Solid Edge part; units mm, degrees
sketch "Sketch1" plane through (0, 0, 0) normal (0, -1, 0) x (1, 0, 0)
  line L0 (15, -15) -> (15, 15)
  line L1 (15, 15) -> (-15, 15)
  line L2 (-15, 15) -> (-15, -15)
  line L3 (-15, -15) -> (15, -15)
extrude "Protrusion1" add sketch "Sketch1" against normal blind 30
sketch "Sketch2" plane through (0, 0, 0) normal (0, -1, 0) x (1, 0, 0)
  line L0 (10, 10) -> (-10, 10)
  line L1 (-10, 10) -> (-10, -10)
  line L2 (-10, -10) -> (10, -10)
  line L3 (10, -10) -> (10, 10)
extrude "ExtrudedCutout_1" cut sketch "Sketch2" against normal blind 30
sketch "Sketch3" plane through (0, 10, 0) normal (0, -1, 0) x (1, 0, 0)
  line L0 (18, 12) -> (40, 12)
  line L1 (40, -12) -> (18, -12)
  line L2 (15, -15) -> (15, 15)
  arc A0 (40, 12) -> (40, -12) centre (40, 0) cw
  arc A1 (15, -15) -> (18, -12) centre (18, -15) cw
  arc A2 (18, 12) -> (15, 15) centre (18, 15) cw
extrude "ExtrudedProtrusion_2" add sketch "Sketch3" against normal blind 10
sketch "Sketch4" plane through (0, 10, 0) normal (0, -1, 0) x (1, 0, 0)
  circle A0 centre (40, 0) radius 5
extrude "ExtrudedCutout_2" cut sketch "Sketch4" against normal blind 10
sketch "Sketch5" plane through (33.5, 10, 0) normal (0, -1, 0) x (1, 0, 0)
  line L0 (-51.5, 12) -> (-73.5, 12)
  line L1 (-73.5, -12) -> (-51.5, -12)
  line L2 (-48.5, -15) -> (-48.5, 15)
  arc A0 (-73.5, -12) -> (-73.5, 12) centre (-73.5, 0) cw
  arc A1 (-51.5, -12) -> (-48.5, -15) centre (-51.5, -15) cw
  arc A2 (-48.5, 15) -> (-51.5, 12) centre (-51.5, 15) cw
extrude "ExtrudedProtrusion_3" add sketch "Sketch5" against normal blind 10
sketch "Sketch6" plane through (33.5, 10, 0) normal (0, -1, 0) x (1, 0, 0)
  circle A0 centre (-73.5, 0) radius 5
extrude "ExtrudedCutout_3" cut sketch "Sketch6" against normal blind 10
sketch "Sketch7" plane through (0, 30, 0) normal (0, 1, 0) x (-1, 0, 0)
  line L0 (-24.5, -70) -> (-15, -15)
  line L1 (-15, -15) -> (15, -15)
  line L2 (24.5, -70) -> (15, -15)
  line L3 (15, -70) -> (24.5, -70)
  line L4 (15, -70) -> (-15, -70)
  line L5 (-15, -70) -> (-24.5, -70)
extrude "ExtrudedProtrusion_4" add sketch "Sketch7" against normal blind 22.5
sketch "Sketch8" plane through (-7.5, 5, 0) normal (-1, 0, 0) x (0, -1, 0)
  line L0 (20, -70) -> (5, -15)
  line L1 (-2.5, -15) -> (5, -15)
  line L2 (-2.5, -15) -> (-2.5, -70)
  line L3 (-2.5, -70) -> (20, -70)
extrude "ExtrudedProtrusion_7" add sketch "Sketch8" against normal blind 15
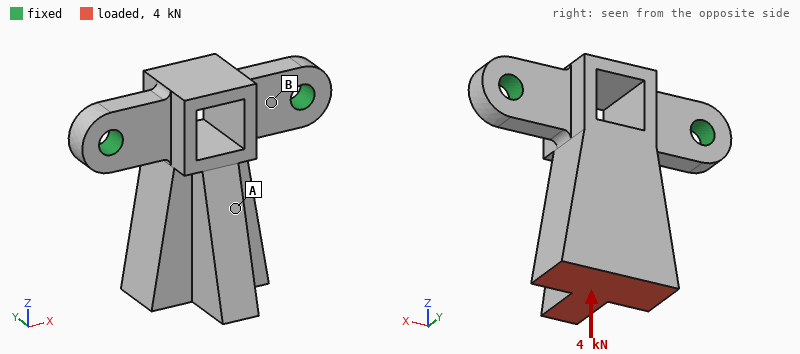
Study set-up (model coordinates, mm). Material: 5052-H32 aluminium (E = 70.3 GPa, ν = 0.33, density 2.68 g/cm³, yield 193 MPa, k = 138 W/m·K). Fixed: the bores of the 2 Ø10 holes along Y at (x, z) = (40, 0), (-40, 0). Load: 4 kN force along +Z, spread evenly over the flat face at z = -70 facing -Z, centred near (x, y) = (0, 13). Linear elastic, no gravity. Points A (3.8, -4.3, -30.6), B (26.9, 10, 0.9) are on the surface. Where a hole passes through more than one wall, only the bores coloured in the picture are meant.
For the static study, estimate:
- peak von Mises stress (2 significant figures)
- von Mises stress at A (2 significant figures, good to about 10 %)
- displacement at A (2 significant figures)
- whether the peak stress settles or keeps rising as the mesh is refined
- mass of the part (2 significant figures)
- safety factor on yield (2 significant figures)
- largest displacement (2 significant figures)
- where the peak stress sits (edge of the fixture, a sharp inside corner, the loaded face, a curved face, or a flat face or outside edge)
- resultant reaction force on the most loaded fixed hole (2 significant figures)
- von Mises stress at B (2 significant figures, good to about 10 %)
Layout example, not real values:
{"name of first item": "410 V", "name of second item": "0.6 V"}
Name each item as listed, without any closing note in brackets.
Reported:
{"peak von Mises stress": "72 MPa", "von Mises stress at A": "5.7 MPa", "displacement at A": "34 µm", "whether the peak stress settles or keeps rising as the mesh is refined": "settles", "mass of the part": "240 g", "safety factor on yield": "2.7", "largest displacement": "56 µm", "where the peak stress sits": "a curved face", "resultant reaction force on the most loaded fixed hole": "2.1 kN", "von Mises stress at B": "28 MPa"}
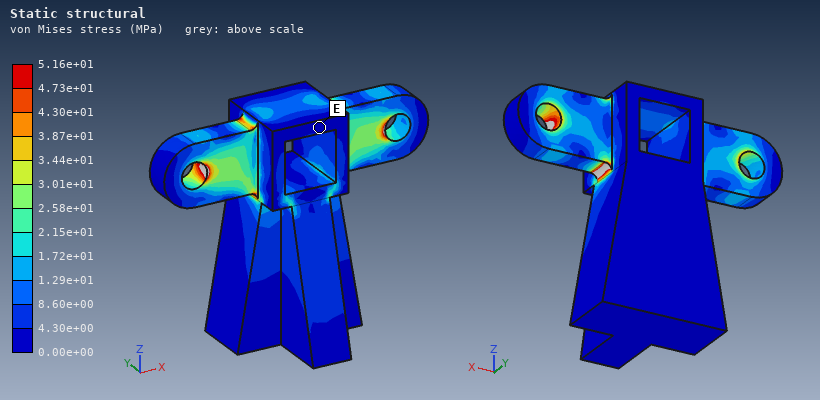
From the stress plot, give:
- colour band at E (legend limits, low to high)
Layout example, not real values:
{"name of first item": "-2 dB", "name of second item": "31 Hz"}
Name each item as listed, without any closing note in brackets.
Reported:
{"colour band at E": "0.00e+00 to 4.30e+00 MPa"}
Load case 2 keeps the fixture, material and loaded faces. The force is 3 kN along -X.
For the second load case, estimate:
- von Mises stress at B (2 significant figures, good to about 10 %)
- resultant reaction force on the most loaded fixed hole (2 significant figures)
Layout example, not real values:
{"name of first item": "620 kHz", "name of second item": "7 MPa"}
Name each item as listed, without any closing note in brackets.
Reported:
{"von Mises stress at B": "41 MPa", "resultant reaction force on the most loaded fixed hole": "4.5 kN"}
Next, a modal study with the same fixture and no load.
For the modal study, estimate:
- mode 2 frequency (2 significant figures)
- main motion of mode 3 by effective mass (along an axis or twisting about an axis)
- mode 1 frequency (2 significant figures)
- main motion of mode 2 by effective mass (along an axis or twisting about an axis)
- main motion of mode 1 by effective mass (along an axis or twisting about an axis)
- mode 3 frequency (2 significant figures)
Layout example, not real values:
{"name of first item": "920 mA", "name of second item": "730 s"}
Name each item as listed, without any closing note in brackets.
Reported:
{"mode 2 frequency": "2200 Hz", "main motion of mode 3 by effective mass": "twisting about Z", "mode 1 frequency": "900 Hz", "main motion of mode 2 by effective mass": "along X", "main motion of mode 1 by effective mass": "along Y", "mode 3 frequency": "4900 Hz"}
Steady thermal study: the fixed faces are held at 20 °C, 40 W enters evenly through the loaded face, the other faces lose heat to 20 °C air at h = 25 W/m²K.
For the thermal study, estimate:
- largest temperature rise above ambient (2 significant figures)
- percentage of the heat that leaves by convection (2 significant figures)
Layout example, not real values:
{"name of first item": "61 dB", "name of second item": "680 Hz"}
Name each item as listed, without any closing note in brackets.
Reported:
{"largest temperature rise above ambient": "33 K", "percentage of the heat that leaves by convection": "20 %"}
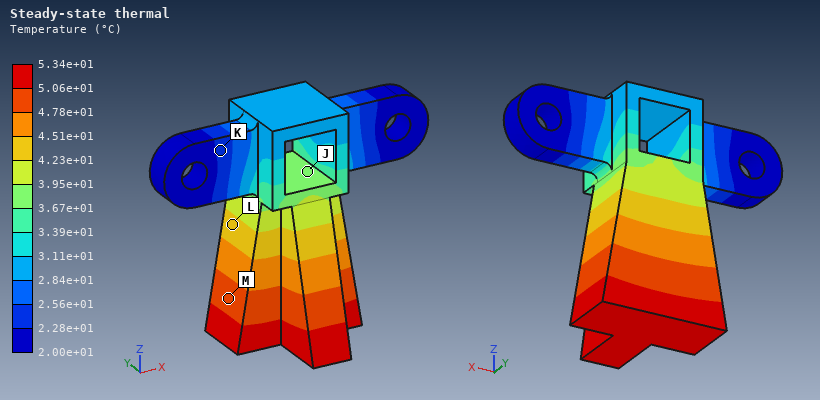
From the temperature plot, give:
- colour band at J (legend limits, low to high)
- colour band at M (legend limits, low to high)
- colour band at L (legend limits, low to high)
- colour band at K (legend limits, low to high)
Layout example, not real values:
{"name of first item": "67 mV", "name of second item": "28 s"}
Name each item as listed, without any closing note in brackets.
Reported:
{"colour band at J": "3.67e+01 to 3.95e+01 °C", "colour band at M": "4.78e+01 to 5.06e+01 °C", "colour band at L": "4.23e+01 to 4.51e+01 °C", "colour band at K": "2.28e+01 to 2.56e+01 °C"}
